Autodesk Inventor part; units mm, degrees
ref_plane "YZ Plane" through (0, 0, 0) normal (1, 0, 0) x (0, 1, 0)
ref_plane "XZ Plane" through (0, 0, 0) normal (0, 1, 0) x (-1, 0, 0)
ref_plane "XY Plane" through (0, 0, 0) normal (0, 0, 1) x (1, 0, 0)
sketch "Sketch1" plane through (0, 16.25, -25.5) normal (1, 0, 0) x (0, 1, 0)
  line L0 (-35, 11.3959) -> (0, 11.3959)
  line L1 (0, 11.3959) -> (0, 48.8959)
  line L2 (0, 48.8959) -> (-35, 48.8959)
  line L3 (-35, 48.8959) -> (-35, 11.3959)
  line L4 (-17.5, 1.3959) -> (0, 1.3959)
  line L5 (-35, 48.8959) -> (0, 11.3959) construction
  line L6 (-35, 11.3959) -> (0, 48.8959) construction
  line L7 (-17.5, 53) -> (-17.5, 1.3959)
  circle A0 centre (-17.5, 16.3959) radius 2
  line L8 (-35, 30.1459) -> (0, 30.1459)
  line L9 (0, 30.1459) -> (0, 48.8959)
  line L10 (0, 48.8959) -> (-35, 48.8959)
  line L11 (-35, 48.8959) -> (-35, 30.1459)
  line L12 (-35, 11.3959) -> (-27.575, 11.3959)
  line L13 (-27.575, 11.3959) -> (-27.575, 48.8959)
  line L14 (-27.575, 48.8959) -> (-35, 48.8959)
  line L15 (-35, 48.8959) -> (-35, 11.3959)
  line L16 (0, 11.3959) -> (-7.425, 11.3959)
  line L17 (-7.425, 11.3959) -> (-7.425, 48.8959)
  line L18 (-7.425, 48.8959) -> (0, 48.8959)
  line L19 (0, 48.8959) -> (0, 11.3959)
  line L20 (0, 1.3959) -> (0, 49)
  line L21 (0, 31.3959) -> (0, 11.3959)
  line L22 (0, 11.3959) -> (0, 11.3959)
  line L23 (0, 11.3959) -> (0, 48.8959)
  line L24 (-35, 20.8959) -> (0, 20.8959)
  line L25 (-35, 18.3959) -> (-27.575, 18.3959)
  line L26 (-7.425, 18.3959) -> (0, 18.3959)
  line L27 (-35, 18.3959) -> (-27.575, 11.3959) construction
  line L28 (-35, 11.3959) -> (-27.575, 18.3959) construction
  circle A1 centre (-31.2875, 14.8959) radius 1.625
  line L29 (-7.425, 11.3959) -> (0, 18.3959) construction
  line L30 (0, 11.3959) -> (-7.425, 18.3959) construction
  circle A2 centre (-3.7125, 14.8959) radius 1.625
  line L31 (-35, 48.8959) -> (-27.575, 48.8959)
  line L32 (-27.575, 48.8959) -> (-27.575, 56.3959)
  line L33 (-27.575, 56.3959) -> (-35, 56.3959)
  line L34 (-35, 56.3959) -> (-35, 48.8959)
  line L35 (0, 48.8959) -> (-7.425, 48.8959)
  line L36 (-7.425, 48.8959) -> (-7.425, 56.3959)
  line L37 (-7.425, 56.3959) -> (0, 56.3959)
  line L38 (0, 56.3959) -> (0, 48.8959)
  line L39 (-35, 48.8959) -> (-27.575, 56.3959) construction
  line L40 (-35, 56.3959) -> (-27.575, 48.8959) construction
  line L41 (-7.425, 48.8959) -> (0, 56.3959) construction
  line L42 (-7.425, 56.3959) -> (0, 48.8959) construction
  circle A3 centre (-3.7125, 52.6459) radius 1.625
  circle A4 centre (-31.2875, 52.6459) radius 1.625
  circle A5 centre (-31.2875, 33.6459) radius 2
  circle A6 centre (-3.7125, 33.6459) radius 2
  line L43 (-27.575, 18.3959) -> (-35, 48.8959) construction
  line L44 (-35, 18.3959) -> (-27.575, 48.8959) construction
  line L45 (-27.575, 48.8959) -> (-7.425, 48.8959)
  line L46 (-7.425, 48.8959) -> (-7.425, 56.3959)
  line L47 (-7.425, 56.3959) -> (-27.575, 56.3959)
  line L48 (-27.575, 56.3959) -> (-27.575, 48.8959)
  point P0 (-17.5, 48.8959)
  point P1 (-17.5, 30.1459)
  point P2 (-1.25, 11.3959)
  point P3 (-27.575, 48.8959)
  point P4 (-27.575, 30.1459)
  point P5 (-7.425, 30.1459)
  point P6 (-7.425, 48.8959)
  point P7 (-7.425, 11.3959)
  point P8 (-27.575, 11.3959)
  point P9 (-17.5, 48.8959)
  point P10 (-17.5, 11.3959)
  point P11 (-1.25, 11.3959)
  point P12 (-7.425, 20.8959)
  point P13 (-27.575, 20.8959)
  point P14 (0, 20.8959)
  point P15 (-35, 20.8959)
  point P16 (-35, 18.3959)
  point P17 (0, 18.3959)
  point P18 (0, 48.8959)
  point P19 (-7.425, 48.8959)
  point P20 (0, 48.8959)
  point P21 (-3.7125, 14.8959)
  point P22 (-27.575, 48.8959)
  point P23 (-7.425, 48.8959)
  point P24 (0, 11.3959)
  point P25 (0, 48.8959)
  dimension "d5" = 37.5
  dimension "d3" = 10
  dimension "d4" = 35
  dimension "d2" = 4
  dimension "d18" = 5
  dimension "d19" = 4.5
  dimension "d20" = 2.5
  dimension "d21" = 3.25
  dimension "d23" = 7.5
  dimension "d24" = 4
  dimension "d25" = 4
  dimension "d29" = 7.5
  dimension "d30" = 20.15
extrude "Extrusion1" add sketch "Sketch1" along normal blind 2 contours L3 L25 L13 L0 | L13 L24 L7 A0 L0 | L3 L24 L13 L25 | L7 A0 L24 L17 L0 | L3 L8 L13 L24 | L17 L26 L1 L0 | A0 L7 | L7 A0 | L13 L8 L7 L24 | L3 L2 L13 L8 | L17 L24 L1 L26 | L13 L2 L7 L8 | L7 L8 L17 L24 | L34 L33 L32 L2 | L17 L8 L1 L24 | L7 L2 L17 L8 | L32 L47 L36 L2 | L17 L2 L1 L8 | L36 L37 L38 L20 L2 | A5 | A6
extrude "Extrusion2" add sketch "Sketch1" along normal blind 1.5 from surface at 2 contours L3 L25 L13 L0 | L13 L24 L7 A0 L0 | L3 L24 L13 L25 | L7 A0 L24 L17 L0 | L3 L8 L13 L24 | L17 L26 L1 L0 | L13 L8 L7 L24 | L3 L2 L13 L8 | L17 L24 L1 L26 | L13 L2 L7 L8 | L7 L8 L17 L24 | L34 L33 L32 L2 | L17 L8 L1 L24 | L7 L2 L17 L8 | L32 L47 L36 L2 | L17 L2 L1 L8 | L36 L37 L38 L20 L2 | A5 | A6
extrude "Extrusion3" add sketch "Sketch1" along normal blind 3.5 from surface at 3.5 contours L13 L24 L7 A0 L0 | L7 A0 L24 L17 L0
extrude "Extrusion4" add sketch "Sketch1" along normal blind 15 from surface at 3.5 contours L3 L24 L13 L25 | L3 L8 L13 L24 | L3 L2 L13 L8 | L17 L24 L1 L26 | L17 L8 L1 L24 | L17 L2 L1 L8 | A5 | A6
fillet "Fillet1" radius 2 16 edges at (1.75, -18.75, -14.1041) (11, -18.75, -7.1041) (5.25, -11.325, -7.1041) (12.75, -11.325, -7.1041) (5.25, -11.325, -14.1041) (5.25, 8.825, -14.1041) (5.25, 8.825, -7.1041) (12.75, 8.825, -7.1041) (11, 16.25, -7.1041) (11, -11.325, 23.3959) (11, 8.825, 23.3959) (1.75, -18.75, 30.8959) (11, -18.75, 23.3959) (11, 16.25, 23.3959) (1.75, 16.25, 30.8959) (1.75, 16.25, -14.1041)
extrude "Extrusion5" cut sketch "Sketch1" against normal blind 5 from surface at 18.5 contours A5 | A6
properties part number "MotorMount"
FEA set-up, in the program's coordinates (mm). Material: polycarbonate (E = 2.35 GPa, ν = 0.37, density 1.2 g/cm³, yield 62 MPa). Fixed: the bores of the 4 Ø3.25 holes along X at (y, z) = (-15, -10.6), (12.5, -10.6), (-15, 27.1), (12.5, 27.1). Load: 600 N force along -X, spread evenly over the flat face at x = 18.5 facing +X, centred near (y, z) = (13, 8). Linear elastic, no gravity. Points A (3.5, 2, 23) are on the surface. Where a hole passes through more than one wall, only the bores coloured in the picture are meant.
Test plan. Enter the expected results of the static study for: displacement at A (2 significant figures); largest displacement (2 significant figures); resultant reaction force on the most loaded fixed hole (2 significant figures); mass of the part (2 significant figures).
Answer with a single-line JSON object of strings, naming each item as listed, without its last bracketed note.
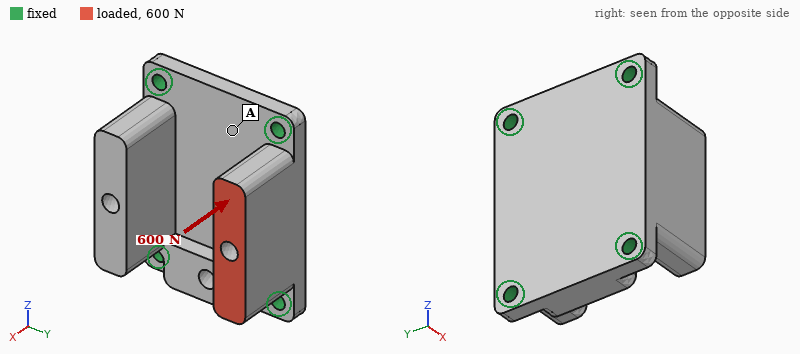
{"displacement at A": "0.036 mm", "largest displacement": "0.19 mm", "resultant reaction force on the most loaded fixed hole": "340 N", "mass of the part": "15 g"}
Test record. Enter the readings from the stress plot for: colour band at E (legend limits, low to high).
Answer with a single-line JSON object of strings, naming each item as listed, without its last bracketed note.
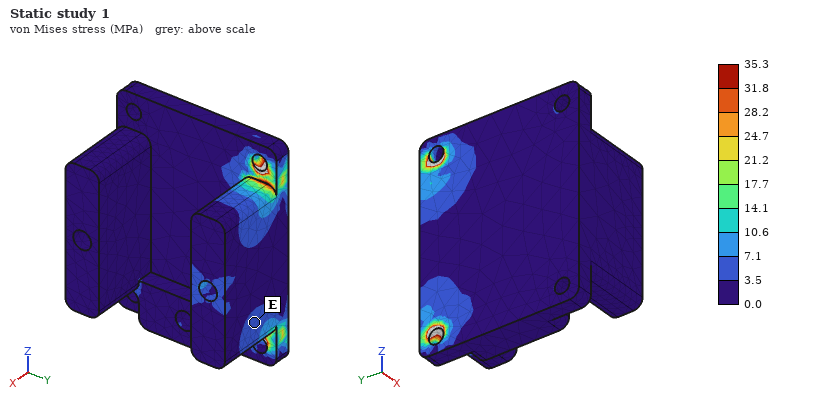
{"colour band at E": "3.5 to 7.1 MPa"}
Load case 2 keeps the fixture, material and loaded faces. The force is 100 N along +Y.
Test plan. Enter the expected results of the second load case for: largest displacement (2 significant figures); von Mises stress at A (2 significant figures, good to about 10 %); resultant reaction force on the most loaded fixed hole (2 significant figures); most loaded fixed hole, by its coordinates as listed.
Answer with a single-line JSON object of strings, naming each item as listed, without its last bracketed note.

{"largest displacement": "0.29 mm", "von Mises stress at A": "3.1 MPa", "resultant reaction force on the most loaded fixed hole": "63 N", "most loaded fixed hole, by its coordinates as listed": "(-15, -10.6)"}
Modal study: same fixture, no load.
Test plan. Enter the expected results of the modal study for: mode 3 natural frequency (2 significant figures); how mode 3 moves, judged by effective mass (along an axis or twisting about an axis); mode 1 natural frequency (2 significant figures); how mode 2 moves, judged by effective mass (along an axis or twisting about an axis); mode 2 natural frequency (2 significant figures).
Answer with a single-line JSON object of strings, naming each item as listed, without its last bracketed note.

{"mode 3 natural frequency": "4400 Hz", "how mode 3 moves, judged by effective mass": "along X", "mode 1 natural frequency": "2300 Hz", "how mode 2 moves, judged by effective mass": "along Y", "mode 2 natural frequency": "2700 Hz"}
